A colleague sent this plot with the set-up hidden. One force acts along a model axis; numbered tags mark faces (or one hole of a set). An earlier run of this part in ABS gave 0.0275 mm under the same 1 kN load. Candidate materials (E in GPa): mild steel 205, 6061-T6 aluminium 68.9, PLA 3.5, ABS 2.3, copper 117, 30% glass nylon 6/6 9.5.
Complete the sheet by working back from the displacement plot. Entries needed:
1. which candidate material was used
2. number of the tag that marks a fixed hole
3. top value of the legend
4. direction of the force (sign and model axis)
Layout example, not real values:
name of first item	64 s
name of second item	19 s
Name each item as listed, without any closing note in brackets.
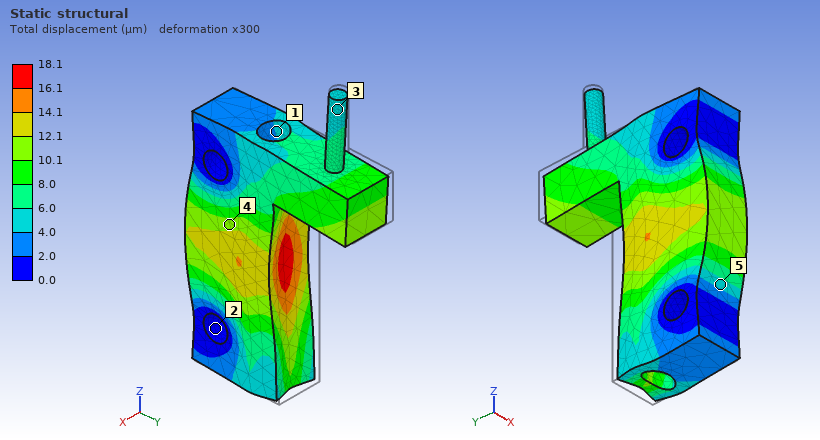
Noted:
which candidate material was used	PLA
number of the tag that marks a fixed hole	2
top value of the legend	18.1 µm
direction of the force	-Y
